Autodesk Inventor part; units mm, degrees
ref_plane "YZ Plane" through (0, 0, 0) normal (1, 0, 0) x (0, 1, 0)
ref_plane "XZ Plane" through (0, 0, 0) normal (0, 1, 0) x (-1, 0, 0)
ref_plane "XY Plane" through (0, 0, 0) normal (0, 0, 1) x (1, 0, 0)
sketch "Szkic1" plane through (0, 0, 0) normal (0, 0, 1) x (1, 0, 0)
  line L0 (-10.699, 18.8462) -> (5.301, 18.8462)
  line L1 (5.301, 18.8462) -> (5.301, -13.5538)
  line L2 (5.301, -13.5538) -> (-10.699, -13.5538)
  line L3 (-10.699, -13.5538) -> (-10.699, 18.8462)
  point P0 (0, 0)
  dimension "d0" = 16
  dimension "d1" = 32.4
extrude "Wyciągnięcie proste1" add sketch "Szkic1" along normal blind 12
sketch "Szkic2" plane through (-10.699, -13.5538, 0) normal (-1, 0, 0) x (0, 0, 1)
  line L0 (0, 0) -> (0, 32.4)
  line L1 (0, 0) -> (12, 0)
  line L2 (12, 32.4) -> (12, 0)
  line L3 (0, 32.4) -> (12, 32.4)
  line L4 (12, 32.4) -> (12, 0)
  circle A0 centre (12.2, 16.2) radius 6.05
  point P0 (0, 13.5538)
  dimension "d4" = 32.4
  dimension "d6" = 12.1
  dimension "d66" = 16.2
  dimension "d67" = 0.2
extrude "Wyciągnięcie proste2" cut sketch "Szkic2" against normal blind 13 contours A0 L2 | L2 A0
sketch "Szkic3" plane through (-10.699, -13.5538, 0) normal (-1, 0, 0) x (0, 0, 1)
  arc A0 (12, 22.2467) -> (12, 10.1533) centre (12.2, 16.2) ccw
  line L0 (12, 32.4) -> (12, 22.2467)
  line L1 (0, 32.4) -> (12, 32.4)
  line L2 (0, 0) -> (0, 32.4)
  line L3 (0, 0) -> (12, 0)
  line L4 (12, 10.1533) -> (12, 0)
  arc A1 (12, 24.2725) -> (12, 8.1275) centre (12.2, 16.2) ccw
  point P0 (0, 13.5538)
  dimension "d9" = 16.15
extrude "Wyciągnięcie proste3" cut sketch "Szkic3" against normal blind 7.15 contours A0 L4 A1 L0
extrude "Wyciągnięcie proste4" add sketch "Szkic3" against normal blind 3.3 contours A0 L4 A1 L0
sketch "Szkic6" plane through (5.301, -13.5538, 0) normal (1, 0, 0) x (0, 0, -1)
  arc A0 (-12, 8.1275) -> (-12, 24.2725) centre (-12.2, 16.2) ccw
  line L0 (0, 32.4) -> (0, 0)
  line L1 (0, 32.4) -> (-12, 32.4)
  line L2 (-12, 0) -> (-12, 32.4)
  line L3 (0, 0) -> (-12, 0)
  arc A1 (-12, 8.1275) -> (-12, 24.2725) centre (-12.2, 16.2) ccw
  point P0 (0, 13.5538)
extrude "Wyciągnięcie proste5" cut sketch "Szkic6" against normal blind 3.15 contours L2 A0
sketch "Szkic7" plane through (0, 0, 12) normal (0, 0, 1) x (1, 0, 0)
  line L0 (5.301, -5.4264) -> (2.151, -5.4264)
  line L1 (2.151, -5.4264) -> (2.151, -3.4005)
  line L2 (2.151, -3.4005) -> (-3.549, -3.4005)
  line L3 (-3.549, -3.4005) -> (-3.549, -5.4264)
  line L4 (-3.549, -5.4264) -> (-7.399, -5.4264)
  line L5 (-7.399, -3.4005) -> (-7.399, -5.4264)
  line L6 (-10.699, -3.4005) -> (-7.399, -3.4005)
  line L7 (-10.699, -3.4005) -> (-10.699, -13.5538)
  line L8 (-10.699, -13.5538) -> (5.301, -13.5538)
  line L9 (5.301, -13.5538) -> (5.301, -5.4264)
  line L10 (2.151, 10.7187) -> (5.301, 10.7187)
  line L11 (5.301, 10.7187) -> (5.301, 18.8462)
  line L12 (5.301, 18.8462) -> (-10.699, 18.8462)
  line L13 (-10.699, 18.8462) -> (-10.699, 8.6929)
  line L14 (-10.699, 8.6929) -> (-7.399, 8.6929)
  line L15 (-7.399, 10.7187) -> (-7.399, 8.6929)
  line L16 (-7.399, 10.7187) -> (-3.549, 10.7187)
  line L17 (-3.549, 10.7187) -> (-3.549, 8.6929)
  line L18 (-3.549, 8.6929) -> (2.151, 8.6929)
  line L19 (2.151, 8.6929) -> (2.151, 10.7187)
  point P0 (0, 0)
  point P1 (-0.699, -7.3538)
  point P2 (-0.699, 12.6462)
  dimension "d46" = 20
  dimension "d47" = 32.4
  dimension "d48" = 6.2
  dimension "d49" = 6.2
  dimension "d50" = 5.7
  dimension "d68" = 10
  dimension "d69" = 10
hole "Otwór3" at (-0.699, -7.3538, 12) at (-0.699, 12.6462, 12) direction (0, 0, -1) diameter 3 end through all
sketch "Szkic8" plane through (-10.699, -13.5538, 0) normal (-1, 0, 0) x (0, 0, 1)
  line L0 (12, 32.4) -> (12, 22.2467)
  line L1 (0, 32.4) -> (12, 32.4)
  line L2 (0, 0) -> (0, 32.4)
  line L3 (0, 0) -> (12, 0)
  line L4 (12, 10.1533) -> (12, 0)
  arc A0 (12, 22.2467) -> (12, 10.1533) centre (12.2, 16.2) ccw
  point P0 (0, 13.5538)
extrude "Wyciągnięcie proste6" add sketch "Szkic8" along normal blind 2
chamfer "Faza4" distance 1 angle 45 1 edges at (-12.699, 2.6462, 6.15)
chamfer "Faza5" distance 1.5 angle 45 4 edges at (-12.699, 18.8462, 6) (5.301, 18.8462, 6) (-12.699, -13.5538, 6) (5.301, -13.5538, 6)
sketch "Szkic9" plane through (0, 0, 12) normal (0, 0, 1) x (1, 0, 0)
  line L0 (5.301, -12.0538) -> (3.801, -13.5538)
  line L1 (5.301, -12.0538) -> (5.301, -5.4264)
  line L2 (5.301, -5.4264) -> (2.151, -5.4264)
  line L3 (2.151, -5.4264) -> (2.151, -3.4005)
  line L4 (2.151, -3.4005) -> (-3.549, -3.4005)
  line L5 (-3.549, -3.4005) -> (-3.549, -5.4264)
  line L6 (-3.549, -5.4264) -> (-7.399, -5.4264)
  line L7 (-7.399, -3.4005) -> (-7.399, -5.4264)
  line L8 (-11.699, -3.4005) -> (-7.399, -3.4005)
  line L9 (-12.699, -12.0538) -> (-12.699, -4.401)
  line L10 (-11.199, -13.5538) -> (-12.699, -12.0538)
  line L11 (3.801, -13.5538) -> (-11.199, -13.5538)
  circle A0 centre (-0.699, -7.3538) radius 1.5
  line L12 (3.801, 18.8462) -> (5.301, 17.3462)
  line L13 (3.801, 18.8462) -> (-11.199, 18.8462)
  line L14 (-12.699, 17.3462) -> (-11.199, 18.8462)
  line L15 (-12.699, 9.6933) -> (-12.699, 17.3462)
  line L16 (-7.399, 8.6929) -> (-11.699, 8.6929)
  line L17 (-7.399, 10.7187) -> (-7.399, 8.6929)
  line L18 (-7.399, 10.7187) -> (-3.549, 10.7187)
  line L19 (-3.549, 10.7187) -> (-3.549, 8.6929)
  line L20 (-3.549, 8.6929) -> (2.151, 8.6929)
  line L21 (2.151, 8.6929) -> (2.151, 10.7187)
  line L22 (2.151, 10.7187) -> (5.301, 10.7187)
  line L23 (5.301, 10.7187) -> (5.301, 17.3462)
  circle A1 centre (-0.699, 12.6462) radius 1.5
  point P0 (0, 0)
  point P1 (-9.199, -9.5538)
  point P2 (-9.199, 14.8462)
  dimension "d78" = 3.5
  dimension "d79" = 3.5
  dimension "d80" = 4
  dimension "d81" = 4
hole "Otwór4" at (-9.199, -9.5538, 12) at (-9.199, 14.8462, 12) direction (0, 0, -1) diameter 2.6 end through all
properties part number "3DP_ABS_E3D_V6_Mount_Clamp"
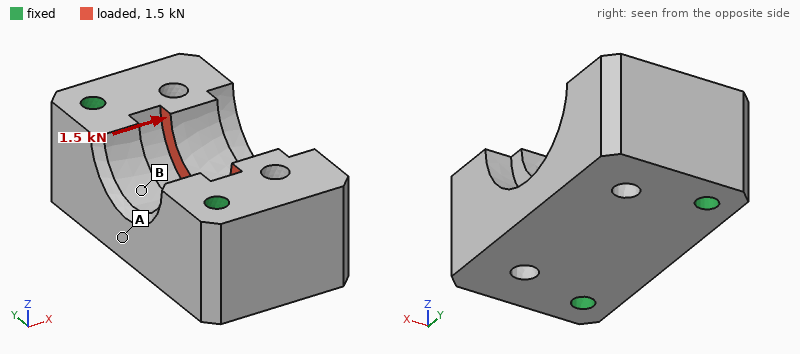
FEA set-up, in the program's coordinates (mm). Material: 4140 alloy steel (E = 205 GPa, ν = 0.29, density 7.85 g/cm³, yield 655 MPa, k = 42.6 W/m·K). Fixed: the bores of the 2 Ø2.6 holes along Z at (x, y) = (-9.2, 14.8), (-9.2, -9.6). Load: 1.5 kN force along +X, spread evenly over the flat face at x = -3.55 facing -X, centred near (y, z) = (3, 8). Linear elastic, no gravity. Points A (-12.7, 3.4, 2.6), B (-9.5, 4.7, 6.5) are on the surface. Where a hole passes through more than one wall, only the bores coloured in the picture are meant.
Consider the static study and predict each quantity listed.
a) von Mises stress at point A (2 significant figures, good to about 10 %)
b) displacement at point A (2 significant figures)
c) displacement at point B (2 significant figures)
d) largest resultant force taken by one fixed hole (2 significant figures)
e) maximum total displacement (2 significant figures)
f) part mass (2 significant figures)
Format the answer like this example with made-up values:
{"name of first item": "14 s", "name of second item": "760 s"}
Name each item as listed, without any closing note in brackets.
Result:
{"von Mises stress at point A": "8.9 MPa", "displacement at point A": "0.70 µm", "displacement at point B": "0.68 µm", "largest resultant force taken by one fixed hole": "810 N", "maximum total displacement": "1.9 µm", "part mass": "42 g"}
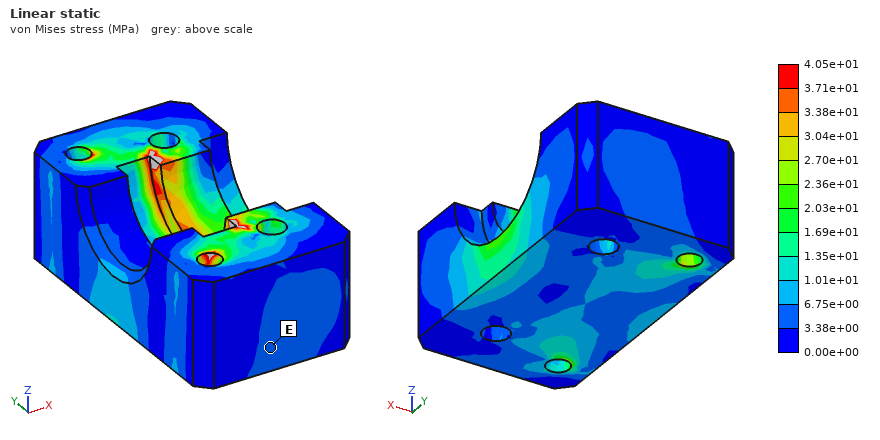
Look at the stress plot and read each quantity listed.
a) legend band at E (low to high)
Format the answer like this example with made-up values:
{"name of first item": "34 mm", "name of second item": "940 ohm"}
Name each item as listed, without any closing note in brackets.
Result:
{"legend band at E": "3.38e+00 to 6.75e+00 MPa"}
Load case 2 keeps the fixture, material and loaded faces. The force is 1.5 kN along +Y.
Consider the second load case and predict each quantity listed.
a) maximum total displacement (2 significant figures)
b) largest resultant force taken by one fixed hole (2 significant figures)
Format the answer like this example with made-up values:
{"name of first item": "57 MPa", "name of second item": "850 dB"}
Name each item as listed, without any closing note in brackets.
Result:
{"maximum total displacement": "1.8 µm", "largest resultant force taken by one fixed hole": "800 N"}
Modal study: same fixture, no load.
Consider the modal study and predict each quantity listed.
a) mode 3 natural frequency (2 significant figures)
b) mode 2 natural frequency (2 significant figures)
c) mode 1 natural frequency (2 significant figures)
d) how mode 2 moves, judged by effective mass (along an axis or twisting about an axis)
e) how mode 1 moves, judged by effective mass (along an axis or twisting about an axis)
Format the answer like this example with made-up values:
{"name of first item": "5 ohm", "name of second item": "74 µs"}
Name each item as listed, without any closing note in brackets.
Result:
{"mode 3 natural frequency": "39 kHz", "mode 2 natural frequency": "33 kHz", "mode 1 natural frequency": "26 kHz", "how mode 2 moves, judged by effective mass": "along Y", "how mode 1 moves, judged by effective mass": "along Z"}
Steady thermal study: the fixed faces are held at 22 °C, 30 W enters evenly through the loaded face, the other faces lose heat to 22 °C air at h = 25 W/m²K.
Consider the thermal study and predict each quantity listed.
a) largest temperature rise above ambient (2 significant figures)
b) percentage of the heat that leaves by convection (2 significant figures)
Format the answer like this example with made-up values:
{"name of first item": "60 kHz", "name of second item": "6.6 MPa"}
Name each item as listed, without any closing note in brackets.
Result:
{"largest temperature rise above ambient": "58 K", "percentage of the heat that leaves by convection": "3.2 %"}
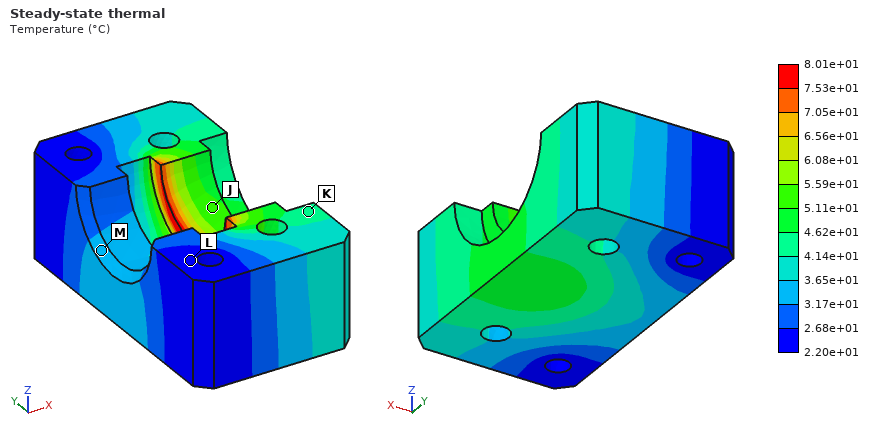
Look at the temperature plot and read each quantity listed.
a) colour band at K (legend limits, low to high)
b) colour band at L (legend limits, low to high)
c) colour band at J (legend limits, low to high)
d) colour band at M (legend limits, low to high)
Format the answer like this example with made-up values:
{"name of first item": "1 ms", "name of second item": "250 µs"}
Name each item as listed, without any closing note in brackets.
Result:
{"colour band at K": "4.14e+01 to 4.62e+01 °C", "colour band at L": "2.20e+01 to 2.68e+01 °C", "colour band at J": "5.11e+01 to 5.59e+01 °C", "colour band at M": "3.17e+01 to 3.65e+01 °C"}
